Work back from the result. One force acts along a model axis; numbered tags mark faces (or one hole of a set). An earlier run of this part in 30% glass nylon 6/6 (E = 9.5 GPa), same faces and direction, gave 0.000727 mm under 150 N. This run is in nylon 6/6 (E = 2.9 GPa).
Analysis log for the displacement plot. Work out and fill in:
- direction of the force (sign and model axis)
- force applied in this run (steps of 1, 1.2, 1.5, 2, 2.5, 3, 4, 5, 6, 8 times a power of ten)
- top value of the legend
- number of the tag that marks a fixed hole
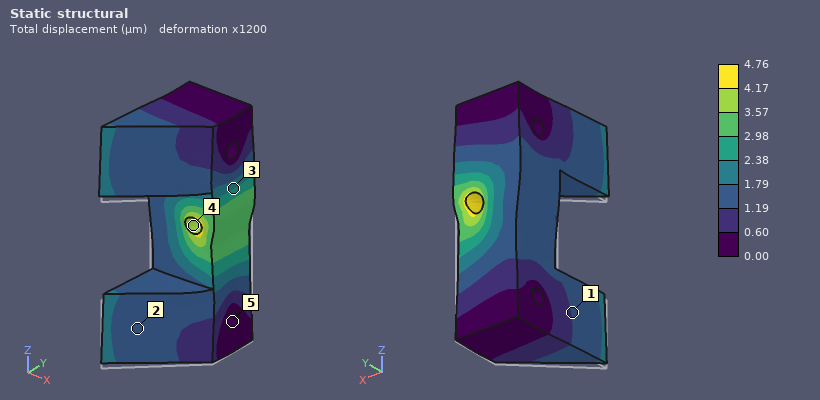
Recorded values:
+Z
300 N
4.76 µm
5
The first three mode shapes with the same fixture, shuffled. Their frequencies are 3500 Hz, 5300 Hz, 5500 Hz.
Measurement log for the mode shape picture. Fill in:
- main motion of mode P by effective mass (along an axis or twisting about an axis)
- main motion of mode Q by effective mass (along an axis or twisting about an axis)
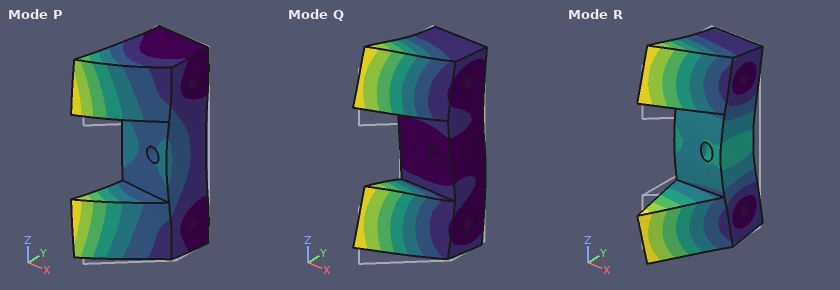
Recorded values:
along X
along Z
